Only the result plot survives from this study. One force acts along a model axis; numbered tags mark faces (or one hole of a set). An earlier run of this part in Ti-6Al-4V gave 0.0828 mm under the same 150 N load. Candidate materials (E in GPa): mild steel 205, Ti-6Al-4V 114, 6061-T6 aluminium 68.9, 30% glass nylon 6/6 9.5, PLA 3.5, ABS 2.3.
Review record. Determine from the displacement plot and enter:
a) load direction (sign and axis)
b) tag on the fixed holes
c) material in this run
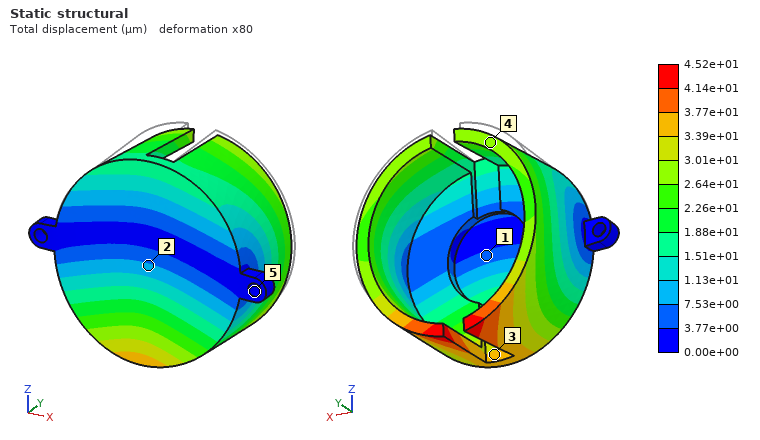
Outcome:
-Y
5
mild steel
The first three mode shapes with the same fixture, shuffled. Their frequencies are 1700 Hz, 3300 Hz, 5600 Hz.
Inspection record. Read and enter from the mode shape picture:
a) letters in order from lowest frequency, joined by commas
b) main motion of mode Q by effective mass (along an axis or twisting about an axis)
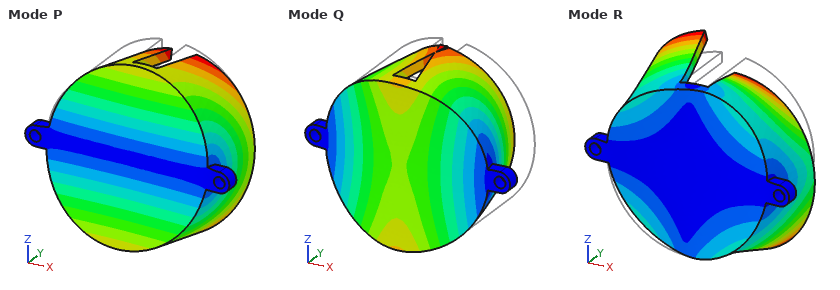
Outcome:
P, Q, R
along Y
